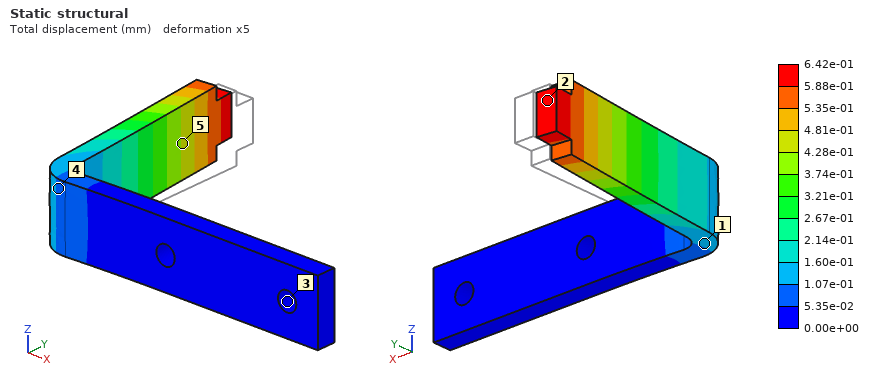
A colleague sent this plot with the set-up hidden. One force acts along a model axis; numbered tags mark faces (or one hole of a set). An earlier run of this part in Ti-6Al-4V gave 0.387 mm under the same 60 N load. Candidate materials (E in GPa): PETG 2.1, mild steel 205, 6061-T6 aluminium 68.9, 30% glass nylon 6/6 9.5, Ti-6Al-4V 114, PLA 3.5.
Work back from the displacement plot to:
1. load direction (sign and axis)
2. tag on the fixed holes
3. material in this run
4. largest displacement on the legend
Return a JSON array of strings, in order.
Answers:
["-X", "3", "6061-T6 aluminium", "6.42e-01 mm"]
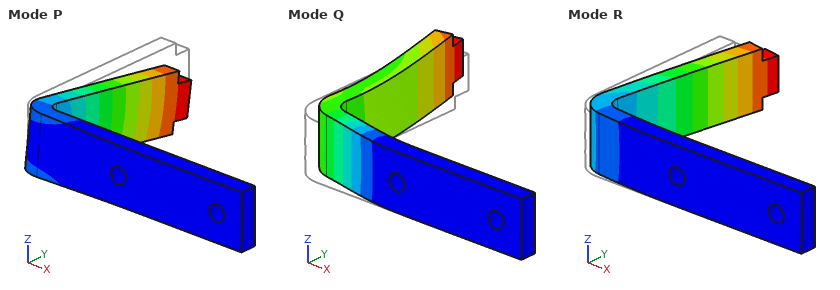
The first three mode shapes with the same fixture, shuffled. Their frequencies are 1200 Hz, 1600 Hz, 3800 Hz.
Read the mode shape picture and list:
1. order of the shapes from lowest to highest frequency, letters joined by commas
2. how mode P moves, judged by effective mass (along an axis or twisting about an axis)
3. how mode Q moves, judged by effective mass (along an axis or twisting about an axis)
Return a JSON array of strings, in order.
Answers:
["R, P, Q", "along Z", "along Y"]
